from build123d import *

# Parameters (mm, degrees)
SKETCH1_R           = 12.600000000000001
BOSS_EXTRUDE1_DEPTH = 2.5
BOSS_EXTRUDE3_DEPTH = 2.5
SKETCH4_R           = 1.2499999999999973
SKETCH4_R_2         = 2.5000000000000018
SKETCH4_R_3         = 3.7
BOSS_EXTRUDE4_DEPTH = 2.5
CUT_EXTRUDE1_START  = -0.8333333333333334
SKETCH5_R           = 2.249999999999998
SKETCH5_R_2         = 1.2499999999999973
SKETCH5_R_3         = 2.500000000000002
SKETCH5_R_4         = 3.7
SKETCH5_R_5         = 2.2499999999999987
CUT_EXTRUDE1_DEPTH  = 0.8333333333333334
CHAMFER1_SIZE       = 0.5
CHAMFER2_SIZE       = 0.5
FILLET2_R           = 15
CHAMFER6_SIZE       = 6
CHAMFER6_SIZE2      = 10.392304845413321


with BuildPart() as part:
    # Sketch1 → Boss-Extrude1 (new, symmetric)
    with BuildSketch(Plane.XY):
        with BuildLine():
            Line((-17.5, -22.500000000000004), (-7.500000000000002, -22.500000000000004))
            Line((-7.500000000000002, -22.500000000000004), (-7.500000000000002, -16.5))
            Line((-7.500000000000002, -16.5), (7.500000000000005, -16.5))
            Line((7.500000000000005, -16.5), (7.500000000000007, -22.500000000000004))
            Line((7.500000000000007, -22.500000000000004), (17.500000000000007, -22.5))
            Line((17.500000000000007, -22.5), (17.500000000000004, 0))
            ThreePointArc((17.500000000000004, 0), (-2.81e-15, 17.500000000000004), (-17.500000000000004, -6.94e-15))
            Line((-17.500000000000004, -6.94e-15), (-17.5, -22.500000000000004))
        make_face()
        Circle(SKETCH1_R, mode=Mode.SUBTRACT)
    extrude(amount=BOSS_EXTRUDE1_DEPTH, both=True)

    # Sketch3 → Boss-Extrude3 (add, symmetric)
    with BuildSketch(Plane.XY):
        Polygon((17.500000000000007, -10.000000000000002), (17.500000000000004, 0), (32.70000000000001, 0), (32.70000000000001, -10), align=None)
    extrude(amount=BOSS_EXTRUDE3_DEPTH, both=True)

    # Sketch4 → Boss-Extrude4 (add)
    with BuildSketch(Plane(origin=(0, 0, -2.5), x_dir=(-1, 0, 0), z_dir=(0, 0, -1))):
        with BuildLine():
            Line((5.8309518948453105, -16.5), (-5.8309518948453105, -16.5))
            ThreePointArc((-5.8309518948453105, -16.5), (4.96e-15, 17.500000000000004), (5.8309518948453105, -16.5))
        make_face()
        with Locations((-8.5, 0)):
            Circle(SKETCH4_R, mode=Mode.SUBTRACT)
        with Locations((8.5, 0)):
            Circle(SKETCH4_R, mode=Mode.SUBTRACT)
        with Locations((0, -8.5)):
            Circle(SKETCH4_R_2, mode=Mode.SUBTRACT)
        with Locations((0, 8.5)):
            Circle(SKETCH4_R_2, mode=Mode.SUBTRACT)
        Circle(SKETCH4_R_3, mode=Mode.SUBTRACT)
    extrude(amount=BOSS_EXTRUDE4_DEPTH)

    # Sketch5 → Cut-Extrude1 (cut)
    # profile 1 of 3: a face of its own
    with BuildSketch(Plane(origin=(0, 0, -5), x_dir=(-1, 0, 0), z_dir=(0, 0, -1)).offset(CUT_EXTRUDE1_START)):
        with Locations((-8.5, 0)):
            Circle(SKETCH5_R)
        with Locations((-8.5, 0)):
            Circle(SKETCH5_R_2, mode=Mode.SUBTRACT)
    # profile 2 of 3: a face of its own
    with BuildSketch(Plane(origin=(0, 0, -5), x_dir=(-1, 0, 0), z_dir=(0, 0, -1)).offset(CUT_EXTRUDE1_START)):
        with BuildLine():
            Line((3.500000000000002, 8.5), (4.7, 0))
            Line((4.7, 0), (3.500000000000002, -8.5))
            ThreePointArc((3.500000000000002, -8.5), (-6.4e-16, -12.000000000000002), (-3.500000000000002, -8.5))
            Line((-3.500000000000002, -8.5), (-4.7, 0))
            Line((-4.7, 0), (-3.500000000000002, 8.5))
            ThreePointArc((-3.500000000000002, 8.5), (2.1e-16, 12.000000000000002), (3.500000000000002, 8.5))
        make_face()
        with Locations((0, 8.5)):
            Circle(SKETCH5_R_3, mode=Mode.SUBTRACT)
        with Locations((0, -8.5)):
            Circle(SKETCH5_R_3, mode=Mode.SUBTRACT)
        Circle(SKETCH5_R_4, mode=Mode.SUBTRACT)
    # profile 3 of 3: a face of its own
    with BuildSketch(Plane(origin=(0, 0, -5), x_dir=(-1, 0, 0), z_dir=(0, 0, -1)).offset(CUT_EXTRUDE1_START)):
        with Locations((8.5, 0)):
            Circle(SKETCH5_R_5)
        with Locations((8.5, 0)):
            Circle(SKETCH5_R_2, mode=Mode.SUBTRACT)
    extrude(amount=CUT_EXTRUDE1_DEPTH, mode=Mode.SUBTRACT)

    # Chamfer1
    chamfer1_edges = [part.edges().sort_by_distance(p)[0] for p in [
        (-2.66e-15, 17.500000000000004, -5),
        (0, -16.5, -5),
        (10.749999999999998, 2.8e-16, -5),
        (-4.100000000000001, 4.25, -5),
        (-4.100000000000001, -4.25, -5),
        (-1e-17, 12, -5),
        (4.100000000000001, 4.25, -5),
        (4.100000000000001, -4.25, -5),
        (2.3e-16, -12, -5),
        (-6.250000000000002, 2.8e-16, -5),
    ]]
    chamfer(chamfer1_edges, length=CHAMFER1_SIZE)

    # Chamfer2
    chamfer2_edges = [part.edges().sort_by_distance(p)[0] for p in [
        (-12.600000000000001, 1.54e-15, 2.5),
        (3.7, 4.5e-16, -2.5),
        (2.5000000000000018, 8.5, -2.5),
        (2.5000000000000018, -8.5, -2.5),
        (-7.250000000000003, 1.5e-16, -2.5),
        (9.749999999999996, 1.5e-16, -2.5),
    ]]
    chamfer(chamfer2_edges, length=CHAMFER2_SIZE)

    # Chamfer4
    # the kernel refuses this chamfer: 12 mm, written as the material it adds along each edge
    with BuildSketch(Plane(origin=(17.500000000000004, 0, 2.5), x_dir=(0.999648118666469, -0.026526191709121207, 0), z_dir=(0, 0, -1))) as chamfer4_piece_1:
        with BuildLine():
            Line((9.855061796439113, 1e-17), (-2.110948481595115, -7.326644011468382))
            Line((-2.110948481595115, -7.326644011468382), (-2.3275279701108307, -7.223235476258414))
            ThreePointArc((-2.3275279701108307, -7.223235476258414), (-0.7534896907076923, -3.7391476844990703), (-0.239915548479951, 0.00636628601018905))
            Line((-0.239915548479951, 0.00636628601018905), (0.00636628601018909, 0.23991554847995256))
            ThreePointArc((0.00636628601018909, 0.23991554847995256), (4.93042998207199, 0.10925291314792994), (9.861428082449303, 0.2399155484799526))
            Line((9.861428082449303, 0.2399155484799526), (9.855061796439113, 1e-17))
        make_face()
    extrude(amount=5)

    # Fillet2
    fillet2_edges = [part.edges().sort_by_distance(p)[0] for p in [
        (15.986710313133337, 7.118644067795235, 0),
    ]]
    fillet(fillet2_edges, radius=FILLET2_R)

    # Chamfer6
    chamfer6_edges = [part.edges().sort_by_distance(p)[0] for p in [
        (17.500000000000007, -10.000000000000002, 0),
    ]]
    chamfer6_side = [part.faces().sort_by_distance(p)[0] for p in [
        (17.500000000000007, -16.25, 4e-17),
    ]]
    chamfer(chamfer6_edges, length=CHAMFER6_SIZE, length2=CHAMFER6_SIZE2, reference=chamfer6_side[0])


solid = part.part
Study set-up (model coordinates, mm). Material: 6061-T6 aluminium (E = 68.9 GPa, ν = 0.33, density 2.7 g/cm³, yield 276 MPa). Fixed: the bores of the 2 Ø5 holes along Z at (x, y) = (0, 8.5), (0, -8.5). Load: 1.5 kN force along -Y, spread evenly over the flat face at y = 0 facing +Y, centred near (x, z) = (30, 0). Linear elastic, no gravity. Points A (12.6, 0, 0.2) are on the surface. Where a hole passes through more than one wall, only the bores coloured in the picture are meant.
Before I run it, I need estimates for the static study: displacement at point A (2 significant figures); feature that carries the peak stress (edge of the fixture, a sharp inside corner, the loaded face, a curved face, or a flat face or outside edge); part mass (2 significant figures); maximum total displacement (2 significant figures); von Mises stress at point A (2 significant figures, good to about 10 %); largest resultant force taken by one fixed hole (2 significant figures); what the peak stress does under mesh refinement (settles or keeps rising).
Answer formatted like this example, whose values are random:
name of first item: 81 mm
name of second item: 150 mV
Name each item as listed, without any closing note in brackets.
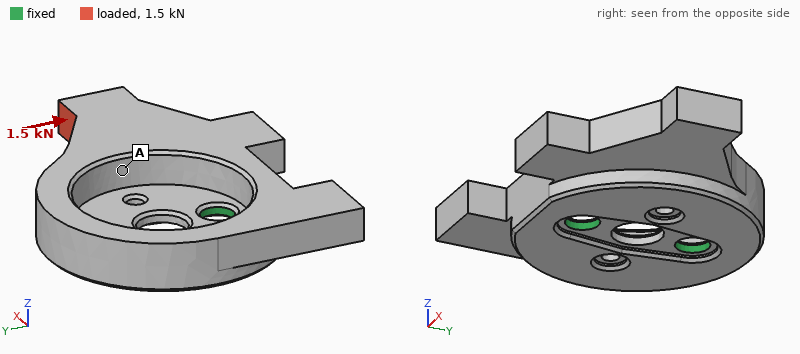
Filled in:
displacement at point A: 24 µm
feature that carries the peak stress: edge of the fixture
part mass: 18 g
maximum total displacement: 87 µm
von Mises stress at point A: 21 MPa
largest resultant force taken by one fixed hole: 2.3 kN
what the peak stress does under mesh refinement: keeps rising
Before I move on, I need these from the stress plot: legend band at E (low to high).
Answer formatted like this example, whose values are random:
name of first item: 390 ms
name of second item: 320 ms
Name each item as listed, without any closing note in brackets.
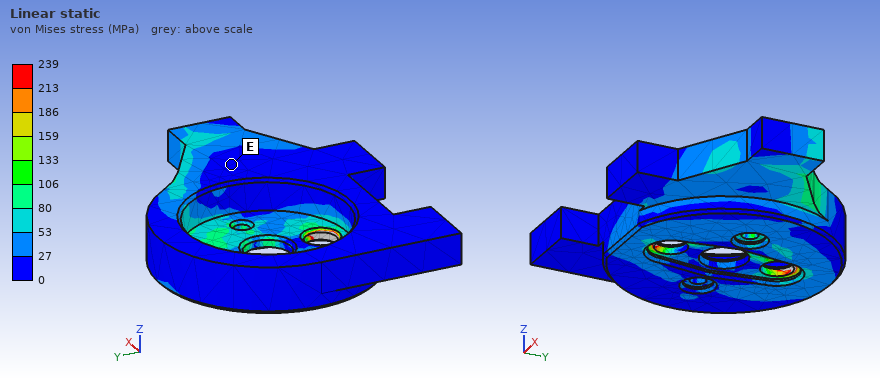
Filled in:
legend band at E: 0 to 27 MPa
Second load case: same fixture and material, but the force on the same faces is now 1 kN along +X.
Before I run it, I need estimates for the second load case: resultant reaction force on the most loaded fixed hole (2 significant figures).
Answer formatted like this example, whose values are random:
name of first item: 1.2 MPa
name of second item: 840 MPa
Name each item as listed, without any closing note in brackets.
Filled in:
resultant reaction force on the most loaded fixed hole: 550 N
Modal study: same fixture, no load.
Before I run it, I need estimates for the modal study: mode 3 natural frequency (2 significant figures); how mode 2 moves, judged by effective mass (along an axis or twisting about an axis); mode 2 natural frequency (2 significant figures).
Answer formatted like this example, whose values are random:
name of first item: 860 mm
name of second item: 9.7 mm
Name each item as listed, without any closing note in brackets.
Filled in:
mode 3 natural frequency: 10 kHz
how mode 2 moves, judged by effective mass: along Z
mode 2 natural frequency: 7600 Hz
